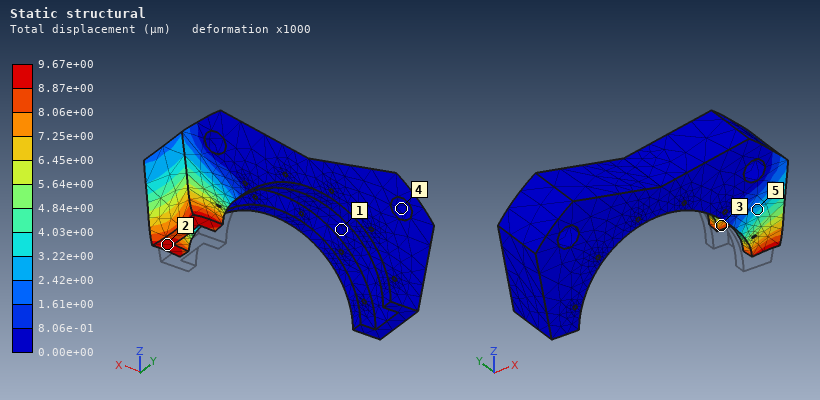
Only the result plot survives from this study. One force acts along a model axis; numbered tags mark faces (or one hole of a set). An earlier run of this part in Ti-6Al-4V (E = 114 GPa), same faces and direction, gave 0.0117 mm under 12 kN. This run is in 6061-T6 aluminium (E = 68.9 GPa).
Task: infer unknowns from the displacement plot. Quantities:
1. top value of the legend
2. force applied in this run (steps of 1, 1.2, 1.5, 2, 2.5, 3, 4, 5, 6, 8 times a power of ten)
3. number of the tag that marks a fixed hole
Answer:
9.67e+00 µm
6 kN
4
